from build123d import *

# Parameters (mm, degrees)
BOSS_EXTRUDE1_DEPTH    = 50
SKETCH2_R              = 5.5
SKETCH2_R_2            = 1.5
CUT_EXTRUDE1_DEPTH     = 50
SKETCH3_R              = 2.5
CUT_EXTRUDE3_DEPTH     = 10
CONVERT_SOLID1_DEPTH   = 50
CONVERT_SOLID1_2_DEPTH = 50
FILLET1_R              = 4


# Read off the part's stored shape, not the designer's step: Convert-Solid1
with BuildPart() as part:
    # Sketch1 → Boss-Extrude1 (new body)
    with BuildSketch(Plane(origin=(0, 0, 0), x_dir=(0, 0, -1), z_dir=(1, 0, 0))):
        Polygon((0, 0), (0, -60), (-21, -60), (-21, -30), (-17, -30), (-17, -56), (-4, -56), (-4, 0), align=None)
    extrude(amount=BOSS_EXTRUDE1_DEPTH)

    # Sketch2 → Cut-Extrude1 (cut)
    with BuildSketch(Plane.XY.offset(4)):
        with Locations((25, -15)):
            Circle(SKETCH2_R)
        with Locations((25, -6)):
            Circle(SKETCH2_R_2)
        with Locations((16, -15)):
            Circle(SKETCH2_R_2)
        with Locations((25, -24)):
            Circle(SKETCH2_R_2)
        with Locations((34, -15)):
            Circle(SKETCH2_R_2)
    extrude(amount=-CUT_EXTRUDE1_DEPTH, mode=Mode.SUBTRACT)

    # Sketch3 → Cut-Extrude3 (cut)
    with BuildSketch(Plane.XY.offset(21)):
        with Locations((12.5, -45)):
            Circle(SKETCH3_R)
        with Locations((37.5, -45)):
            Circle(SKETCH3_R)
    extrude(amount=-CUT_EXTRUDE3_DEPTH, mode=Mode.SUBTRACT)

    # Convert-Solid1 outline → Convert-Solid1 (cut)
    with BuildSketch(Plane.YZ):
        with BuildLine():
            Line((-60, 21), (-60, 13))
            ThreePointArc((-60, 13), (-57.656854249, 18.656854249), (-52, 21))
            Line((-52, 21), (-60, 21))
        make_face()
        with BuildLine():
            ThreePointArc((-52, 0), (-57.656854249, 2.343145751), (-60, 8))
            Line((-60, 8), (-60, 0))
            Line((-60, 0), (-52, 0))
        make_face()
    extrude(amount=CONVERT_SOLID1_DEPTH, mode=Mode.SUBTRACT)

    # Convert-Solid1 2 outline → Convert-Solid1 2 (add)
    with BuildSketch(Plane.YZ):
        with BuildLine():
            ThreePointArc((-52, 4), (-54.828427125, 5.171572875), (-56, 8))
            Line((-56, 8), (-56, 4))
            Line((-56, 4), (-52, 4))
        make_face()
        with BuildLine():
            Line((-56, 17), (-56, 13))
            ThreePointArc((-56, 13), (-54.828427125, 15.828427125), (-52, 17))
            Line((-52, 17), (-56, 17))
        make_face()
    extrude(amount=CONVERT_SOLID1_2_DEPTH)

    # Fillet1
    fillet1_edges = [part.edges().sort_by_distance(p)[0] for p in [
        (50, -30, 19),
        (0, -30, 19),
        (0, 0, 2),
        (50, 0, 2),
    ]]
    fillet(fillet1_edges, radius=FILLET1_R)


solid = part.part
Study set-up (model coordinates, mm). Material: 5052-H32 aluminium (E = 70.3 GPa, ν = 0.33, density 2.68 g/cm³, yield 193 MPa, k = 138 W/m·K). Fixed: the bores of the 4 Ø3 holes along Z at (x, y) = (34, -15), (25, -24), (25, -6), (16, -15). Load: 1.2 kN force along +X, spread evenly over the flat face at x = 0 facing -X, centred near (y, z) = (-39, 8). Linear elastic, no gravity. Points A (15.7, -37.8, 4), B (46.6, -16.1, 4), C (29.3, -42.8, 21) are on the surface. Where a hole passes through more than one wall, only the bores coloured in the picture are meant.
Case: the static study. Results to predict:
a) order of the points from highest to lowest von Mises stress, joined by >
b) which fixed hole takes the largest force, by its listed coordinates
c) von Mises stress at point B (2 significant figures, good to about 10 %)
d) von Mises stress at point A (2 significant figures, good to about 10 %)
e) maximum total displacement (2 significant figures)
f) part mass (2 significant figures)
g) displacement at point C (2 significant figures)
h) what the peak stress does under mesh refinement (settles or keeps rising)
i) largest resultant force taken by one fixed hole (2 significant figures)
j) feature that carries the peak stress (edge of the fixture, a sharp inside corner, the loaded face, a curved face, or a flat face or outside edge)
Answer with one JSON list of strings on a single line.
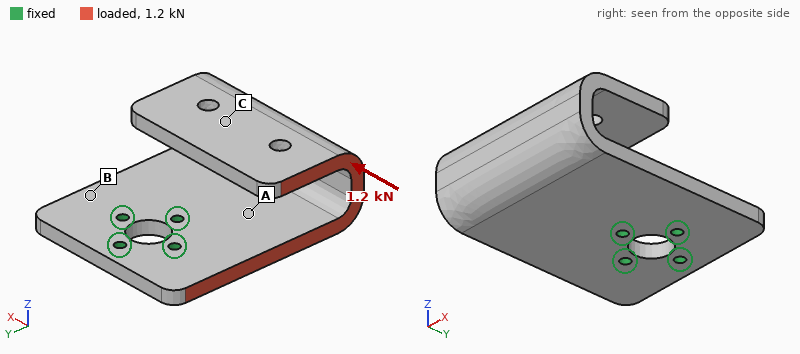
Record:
["A > B > C", "(25, -24)", "20 MPa", "46 MPa", "0.28 mm", "51 g", "0.20 mm", "keeps rising", "1.2 kN", "edge of the fixture"]
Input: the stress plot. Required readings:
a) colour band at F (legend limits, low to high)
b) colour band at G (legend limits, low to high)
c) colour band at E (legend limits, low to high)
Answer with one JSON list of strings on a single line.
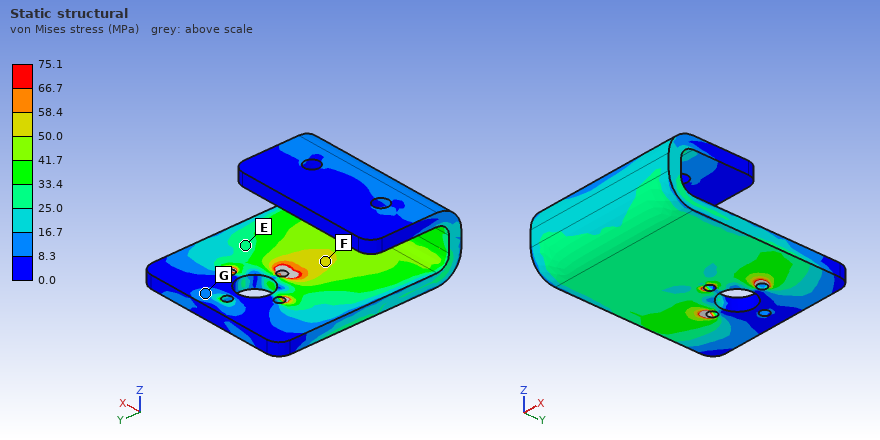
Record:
["50.0 to 58.4 MPa", "8.3 to 16.7 MPa", "25.0 to 33.4 MPa"]
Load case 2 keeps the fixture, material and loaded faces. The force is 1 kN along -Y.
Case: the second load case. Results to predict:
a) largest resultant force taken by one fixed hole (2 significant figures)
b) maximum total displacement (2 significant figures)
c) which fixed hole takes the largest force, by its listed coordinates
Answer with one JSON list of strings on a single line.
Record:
["1.1 kN", "0.35 mm", "(16, -15)"]
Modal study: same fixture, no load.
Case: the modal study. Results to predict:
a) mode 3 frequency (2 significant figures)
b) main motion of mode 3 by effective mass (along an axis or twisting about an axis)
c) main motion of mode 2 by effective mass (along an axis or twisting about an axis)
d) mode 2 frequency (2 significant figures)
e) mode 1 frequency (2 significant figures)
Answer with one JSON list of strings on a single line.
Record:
["1900 Hz", "along Z", "along X", "1400 Hz", "1100 Hz"]
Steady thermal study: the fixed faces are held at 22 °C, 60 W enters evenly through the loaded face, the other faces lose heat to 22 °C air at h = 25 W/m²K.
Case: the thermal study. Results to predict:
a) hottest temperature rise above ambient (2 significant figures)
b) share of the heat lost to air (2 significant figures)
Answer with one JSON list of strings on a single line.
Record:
["76 K", "15 %"]
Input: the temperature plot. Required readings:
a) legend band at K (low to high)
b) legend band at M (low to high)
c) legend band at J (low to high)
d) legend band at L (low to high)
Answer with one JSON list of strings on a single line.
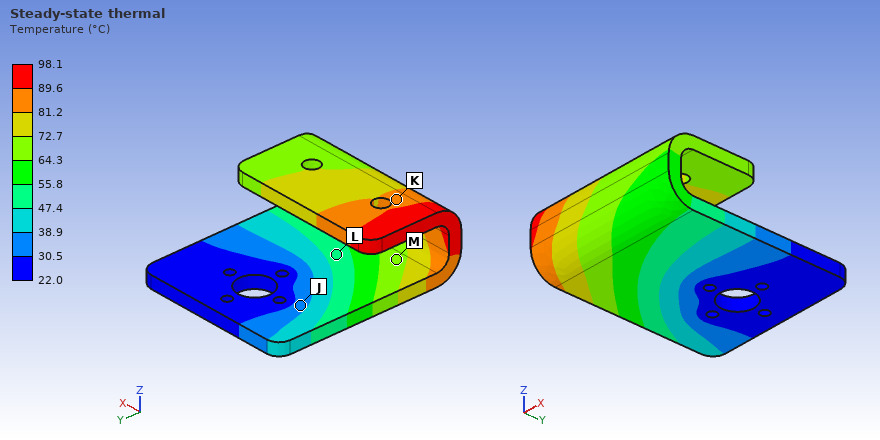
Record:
["81.2 to 89.6 °C", "64.3 to 72.7 °C", "30.5 to 38.9 °C", "47.4 to 55.8 °C"]
